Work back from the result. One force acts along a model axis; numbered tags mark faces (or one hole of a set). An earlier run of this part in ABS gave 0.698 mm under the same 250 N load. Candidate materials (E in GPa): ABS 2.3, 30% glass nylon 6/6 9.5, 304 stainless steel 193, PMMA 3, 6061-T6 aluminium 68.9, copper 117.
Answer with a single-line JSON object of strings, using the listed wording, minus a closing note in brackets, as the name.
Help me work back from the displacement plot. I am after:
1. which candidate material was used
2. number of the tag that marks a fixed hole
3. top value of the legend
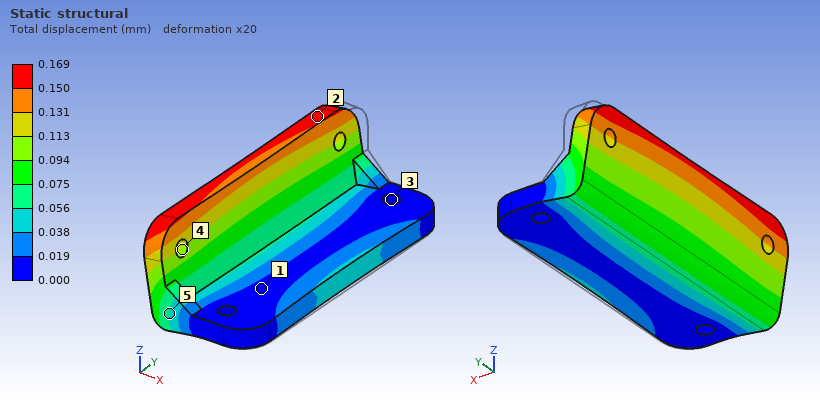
{"which candidate material was used": "30% glass nylon 6/6", "number of the tag that marks a fixed hole": "3", "top value of the legend": "0.169 mm"}
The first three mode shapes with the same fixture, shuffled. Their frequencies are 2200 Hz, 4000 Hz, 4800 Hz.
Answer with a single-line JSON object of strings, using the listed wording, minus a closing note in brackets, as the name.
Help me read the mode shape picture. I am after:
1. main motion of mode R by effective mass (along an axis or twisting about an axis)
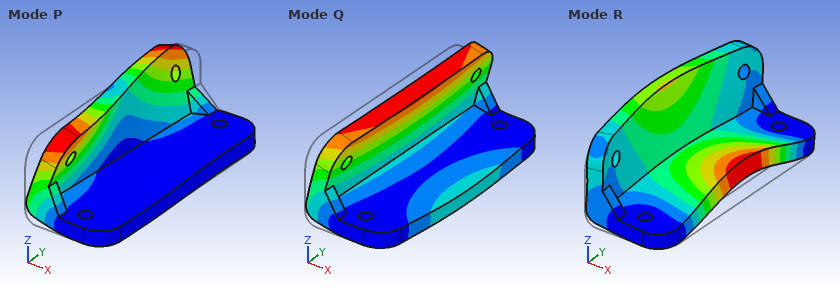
{"main motion of mode R by effective mass": "along Z"}
